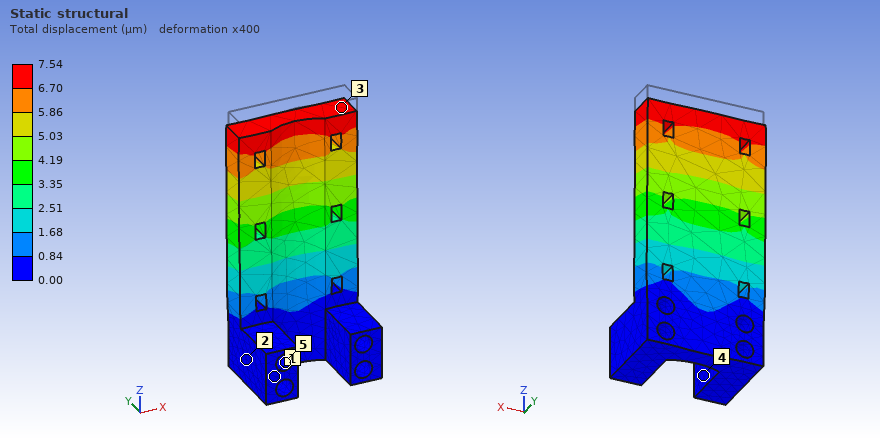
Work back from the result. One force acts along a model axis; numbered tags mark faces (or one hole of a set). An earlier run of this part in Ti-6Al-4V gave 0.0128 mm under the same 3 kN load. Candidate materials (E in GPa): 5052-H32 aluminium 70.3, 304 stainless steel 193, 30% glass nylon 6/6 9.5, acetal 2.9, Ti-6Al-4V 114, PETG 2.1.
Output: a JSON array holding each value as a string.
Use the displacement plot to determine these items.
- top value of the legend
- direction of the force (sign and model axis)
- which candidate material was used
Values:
["7.54 µm", "-Z", "304 stainless steel"]
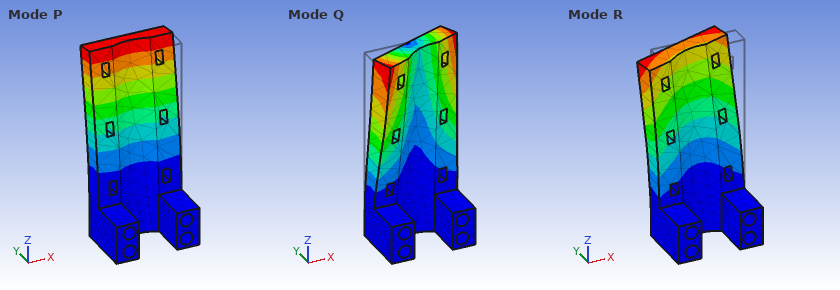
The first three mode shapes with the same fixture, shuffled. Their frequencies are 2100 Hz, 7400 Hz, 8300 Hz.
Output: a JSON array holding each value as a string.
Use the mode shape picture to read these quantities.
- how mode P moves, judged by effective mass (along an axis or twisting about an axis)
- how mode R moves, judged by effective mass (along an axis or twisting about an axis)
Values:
["along Y", "along X"]
